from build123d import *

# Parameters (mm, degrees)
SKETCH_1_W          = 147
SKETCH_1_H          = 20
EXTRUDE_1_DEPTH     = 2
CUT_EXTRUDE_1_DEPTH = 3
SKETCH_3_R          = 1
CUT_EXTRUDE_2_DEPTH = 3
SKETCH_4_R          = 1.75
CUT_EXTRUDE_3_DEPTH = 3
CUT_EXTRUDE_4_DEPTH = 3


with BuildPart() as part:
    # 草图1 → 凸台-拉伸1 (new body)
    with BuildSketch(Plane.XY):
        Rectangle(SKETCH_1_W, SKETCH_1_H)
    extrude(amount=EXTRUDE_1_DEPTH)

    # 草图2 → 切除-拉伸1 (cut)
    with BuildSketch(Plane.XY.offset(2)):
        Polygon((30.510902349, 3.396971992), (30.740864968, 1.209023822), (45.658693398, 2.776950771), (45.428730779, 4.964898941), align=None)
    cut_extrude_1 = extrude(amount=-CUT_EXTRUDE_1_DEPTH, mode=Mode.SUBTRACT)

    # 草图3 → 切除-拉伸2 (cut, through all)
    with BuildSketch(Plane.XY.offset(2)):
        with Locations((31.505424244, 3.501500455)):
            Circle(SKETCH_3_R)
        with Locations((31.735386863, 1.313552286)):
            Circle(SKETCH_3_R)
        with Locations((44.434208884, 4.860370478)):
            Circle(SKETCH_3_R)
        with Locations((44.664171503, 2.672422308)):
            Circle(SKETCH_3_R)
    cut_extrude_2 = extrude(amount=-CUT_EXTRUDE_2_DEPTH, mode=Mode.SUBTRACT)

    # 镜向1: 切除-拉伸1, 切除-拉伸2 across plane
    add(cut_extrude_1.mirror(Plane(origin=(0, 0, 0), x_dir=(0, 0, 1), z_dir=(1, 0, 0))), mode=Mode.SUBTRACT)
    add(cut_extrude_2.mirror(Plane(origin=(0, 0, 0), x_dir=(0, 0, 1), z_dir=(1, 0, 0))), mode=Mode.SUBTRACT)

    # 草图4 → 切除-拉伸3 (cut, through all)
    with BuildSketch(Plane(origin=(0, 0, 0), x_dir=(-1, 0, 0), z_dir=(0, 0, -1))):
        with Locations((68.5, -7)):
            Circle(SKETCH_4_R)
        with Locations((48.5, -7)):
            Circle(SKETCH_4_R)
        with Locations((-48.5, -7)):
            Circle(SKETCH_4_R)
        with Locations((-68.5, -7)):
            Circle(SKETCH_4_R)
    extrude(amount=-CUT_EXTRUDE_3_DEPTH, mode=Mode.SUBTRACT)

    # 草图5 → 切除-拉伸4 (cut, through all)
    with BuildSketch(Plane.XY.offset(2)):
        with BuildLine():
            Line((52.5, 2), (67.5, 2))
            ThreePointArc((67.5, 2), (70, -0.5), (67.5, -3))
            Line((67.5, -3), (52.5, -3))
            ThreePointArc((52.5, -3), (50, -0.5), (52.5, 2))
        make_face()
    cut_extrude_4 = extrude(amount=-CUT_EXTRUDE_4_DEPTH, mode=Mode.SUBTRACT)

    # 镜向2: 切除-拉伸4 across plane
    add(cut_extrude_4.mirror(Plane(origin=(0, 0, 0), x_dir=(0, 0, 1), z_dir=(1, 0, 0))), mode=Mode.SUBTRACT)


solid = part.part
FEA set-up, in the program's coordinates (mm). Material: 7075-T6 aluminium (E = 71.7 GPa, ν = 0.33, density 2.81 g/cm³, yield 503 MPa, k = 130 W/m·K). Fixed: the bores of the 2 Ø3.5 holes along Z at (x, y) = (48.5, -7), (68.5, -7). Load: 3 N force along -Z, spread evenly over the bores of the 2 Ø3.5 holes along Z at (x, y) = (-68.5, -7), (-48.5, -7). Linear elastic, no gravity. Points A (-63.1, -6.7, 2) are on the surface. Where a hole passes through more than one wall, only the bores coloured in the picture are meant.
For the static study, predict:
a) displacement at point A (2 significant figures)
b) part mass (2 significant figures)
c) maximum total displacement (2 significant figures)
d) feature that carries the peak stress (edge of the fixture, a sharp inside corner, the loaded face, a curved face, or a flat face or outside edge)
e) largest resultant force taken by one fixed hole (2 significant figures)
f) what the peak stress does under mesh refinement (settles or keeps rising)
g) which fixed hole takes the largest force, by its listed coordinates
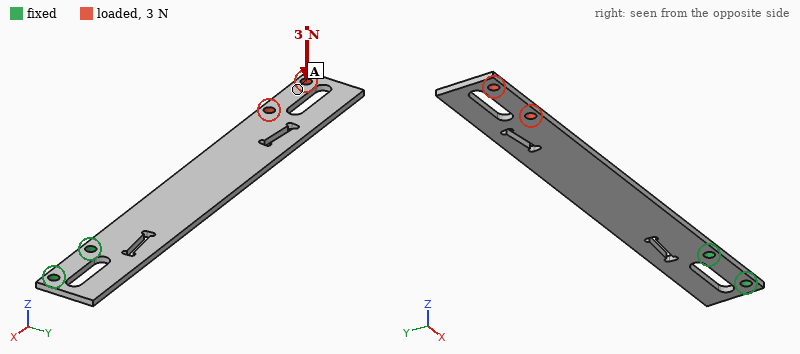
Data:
1.5 mm
15 g
1.7 mm
edge of the fixture
6.5 N
keeps rising
(48.5, -7)
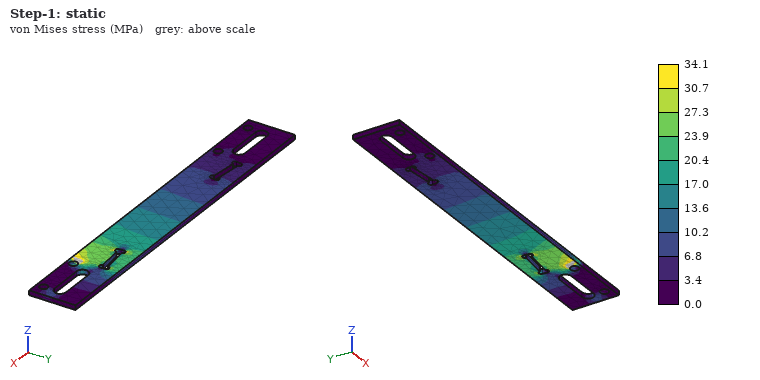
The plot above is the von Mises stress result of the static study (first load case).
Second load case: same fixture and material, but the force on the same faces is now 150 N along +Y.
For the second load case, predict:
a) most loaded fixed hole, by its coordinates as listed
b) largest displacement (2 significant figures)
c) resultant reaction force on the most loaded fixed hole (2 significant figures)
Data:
(48.5, -7)
1.3 mm
740 N
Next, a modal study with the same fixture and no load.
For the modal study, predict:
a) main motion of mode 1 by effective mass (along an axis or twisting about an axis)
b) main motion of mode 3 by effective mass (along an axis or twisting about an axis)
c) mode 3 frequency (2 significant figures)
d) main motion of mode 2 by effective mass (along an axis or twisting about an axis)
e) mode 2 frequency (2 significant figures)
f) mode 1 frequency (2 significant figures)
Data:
along Z
along Y
860 Hz
along Z
670 Hz
110 Hz
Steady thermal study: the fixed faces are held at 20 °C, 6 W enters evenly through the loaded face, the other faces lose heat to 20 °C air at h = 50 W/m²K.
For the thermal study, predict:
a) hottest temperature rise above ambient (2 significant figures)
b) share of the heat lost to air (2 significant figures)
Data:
55 K
86 %
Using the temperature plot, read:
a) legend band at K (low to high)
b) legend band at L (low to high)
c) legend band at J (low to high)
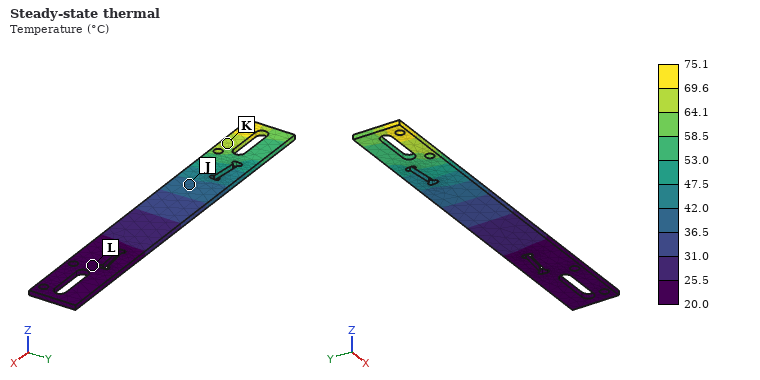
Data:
64.1 to 69.6 °C
20.0 to 25.5 °C
36.5 to 42.0 °C
